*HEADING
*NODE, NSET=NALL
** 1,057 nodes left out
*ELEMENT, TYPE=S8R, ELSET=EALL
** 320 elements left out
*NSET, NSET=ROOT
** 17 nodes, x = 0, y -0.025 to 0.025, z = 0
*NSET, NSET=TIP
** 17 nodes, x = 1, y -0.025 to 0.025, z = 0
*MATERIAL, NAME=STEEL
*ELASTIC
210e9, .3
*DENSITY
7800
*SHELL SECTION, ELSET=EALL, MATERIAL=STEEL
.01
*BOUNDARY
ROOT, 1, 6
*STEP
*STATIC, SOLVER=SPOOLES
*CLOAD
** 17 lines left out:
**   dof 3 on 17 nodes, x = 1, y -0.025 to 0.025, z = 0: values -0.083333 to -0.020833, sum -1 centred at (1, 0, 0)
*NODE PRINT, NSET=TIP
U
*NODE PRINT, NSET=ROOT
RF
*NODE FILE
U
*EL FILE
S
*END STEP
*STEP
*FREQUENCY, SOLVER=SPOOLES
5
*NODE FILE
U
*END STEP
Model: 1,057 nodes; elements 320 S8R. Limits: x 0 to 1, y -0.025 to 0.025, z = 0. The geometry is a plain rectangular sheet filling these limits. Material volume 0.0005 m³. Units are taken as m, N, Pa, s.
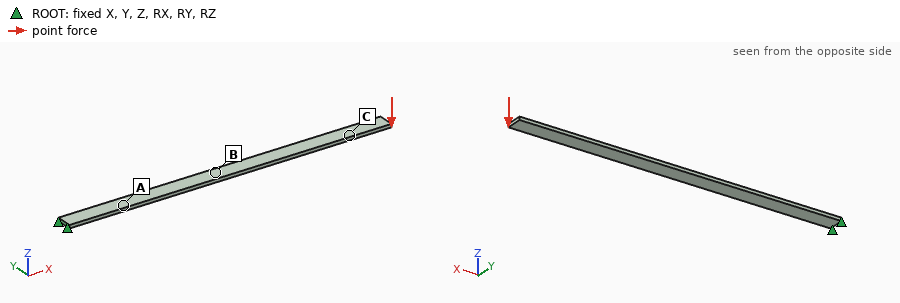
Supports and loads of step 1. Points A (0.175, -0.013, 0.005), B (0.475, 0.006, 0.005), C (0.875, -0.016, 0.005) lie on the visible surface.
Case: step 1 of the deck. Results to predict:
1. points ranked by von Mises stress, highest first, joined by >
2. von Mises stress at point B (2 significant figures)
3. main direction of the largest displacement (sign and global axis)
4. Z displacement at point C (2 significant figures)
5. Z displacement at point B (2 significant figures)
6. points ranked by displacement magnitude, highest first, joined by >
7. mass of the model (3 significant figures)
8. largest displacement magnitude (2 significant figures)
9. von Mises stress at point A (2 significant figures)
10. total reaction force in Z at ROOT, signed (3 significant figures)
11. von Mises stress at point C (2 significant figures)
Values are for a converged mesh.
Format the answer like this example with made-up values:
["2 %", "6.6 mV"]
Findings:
["A > B > C", "6.3e+05 Pa", "-Z", "-3.1e-04 m", "-1.1e-04 m", "C > B > A", "3.90 kg", "3.8e-04 m", "9.9e+05 Pa", "1.00 N", "1.5e+05 Pa"]
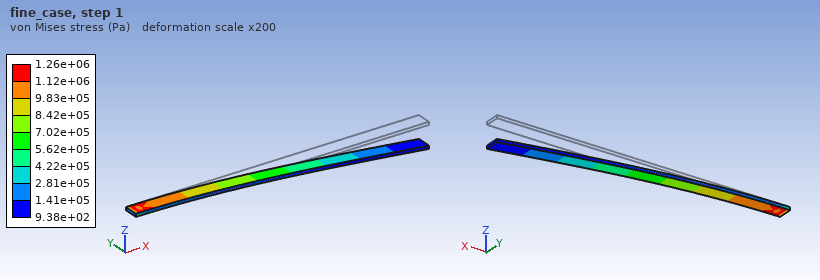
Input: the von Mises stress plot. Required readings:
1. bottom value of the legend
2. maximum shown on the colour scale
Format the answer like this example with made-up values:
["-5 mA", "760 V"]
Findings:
["9.38e+02 Pa", "1.26e+06 Pa"]
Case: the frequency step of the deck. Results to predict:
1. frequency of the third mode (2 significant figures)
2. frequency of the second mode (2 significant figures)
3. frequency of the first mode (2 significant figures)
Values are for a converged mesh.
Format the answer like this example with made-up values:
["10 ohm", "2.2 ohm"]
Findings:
["53 Hz", "42 Hz", "8.4 Hz"]
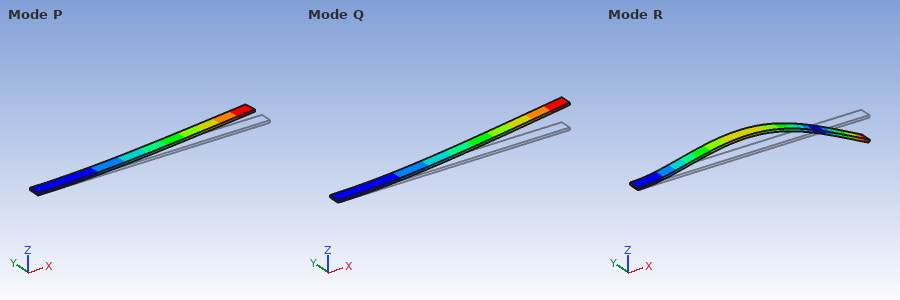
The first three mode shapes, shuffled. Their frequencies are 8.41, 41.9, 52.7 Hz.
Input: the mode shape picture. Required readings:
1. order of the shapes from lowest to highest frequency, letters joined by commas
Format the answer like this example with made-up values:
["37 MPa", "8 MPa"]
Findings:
["Q, P, R"]
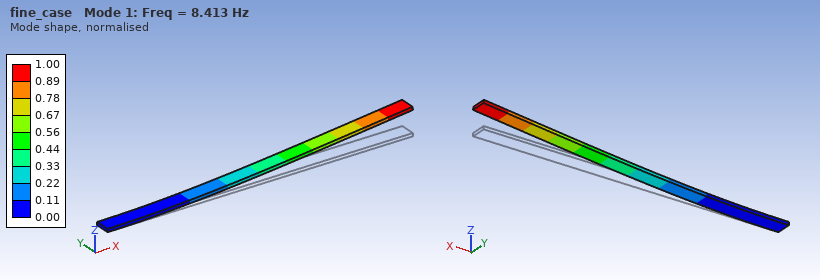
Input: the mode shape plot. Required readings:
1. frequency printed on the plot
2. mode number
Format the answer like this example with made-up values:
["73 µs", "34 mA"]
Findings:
["8.413 Hz", "1"]
